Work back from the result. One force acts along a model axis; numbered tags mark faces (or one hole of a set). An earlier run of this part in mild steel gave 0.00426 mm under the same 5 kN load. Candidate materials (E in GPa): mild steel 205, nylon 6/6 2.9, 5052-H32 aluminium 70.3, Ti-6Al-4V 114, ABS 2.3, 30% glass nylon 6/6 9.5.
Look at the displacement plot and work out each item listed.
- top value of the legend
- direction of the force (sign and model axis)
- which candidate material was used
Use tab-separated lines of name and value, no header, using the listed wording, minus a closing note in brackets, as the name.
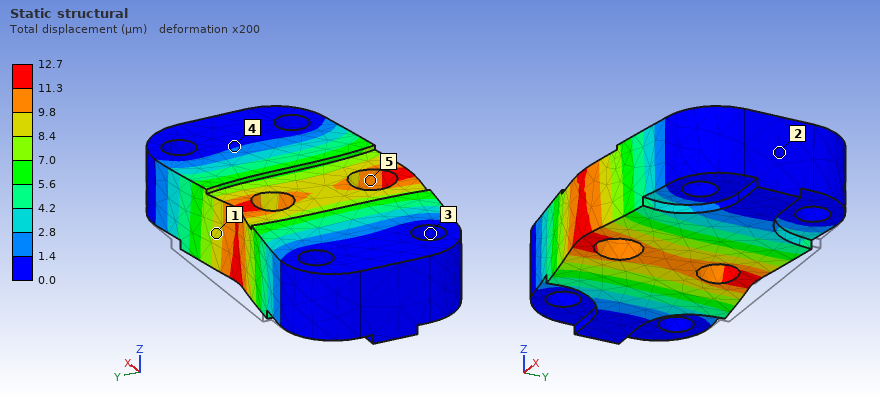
top value of the legend	12.7 µm
direction of the force	-Y
which candidate material was used	5052-H32 aluminium
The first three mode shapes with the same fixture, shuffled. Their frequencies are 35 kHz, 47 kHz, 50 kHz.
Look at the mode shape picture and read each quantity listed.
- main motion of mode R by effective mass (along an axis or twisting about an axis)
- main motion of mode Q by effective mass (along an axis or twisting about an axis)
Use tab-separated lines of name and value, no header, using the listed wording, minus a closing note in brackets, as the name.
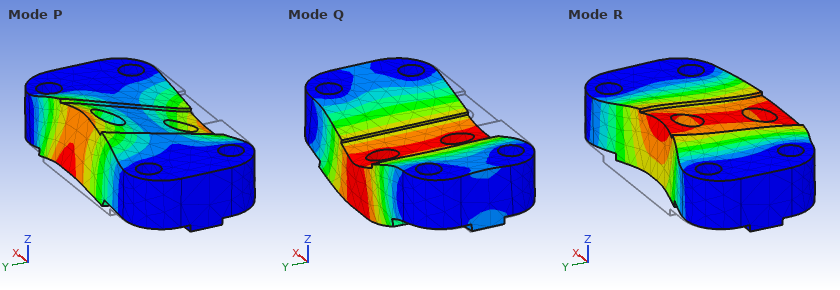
main motion of mode R by effective mass	along Y
main motion of mode Q by effective mass	along Z
